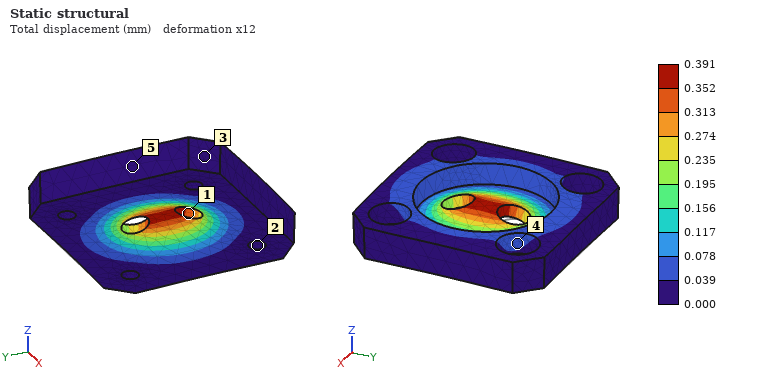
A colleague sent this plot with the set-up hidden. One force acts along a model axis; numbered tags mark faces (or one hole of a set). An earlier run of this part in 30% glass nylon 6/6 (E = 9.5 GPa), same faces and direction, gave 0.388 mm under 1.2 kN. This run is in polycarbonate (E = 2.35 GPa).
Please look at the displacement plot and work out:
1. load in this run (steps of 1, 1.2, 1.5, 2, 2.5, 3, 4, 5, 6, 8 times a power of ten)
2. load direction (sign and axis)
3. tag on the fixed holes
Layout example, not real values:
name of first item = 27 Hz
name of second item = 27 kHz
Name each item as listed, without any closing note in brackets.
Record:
load in this run = 300 N
load direction = +Z
tag on the fixed holes = 2
